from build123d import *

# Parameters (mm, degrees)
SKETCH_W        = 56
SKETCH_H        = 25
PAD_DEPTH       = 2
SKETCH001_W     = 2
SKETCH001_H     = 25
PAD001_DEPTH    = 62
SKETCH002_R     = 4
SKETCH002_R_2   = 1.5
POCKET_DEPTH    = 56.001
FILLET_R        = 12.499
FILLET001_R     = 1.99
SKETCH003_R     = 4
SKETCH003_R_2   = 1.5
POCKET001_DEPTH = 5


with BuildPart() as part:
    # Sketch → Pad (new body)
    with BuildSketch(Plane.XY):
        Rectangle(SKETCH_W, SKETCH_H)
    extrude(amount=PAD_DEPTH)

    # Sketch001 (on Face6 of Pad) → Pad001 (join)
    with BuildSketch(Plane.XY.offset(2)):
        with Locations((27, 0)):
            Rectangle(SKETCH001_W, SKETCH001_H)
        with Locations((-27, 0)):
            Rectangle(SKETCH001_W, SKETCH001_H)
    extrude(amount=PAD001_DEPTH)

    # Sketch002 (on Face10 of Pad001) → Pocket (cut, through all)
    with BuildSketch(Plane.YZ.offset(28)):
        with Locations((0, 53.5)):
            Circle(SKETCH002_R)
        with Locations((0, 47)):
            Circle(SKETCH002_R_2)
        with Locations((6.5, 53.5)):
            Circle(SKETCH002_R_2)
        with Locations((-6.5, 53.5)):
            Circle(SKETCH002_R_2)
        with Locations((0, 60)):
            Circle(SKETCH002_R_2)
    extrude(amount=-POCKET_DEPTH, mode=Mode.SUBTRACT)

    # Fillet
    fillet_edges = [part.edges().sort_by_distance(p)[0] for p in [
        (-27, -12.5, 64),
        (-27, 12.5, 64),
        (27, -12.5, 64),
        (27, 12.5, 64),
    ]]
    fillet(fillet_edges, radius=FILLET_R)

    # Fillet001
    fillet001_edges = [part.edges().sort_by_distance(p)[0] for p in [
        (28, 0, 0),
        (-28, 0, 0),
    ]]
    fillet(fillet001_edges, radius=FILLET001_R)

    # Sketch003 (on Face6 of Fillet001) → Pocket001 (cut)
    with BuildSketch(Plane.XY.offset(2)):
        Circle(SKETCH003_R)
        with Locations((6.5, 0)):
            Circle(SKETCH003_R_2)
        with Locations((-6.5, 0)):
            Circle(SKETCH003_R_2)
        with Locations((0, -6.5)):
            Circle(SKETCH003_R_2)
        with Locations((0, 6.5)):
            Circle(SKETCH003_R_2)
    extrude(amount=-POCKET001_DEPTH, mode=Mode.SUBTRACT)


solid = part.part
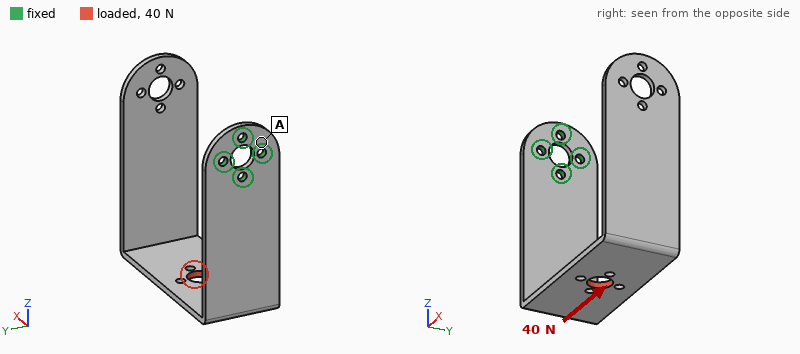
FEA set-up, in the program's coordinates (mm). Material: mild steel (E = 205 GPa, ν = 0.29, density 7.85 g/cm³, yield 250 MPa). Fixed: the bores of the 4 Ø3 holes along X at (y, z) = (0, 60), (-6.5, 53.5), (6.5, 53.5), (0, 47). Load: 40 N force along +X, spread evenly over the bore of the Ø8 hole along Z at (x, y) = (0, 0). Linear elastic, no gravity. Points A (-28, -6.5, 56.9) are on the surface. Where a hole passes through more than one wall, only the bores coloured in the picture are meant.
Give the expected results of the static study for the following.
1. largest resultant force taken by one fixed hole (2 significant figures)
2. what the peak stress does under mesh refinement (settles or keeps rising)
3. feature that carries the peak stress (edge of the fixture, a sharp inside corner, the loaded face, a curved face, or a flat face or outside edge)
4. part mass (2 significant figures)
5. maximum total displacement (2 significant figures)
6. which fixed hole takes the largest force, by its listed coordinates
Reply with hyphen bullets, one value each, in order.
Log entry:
- 170 N
- keeps rising
- edge of the fixture
- 65 g
- 0.77 mm
- (0, 47)
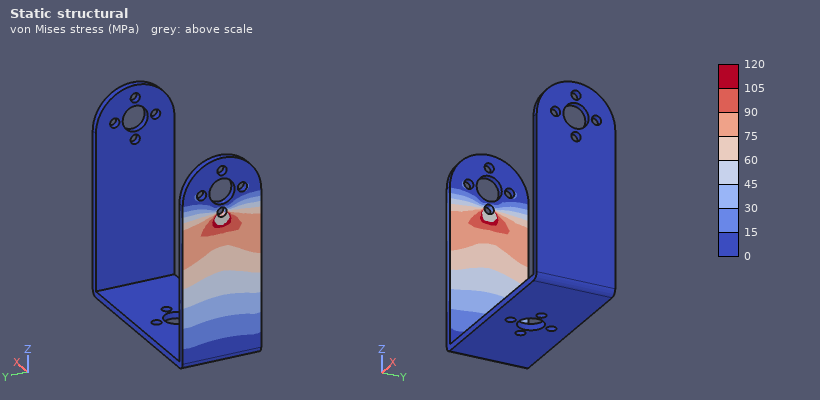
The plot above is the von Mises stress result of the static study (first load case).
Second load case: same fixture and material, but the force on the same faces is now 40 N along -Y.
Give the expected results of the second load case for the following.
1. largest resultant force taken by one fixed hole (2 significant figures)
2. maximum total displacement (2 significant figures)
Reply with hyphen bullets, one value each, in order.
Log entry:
- 97 N
- 0.54 mm
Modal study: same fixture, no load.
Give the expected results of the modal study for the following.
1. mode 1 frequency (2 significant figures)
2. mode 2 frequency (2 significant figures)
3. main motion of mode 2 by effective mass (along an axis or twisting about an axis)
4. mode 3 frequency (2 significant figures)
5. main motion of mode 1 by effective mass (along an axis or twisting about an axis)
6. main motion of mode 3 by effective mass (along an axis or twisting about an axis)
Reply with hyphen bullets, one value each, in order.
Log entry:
- 110 Hz
- 160 Hz
- along Y
- 250 Hz
- along Z
- along X
